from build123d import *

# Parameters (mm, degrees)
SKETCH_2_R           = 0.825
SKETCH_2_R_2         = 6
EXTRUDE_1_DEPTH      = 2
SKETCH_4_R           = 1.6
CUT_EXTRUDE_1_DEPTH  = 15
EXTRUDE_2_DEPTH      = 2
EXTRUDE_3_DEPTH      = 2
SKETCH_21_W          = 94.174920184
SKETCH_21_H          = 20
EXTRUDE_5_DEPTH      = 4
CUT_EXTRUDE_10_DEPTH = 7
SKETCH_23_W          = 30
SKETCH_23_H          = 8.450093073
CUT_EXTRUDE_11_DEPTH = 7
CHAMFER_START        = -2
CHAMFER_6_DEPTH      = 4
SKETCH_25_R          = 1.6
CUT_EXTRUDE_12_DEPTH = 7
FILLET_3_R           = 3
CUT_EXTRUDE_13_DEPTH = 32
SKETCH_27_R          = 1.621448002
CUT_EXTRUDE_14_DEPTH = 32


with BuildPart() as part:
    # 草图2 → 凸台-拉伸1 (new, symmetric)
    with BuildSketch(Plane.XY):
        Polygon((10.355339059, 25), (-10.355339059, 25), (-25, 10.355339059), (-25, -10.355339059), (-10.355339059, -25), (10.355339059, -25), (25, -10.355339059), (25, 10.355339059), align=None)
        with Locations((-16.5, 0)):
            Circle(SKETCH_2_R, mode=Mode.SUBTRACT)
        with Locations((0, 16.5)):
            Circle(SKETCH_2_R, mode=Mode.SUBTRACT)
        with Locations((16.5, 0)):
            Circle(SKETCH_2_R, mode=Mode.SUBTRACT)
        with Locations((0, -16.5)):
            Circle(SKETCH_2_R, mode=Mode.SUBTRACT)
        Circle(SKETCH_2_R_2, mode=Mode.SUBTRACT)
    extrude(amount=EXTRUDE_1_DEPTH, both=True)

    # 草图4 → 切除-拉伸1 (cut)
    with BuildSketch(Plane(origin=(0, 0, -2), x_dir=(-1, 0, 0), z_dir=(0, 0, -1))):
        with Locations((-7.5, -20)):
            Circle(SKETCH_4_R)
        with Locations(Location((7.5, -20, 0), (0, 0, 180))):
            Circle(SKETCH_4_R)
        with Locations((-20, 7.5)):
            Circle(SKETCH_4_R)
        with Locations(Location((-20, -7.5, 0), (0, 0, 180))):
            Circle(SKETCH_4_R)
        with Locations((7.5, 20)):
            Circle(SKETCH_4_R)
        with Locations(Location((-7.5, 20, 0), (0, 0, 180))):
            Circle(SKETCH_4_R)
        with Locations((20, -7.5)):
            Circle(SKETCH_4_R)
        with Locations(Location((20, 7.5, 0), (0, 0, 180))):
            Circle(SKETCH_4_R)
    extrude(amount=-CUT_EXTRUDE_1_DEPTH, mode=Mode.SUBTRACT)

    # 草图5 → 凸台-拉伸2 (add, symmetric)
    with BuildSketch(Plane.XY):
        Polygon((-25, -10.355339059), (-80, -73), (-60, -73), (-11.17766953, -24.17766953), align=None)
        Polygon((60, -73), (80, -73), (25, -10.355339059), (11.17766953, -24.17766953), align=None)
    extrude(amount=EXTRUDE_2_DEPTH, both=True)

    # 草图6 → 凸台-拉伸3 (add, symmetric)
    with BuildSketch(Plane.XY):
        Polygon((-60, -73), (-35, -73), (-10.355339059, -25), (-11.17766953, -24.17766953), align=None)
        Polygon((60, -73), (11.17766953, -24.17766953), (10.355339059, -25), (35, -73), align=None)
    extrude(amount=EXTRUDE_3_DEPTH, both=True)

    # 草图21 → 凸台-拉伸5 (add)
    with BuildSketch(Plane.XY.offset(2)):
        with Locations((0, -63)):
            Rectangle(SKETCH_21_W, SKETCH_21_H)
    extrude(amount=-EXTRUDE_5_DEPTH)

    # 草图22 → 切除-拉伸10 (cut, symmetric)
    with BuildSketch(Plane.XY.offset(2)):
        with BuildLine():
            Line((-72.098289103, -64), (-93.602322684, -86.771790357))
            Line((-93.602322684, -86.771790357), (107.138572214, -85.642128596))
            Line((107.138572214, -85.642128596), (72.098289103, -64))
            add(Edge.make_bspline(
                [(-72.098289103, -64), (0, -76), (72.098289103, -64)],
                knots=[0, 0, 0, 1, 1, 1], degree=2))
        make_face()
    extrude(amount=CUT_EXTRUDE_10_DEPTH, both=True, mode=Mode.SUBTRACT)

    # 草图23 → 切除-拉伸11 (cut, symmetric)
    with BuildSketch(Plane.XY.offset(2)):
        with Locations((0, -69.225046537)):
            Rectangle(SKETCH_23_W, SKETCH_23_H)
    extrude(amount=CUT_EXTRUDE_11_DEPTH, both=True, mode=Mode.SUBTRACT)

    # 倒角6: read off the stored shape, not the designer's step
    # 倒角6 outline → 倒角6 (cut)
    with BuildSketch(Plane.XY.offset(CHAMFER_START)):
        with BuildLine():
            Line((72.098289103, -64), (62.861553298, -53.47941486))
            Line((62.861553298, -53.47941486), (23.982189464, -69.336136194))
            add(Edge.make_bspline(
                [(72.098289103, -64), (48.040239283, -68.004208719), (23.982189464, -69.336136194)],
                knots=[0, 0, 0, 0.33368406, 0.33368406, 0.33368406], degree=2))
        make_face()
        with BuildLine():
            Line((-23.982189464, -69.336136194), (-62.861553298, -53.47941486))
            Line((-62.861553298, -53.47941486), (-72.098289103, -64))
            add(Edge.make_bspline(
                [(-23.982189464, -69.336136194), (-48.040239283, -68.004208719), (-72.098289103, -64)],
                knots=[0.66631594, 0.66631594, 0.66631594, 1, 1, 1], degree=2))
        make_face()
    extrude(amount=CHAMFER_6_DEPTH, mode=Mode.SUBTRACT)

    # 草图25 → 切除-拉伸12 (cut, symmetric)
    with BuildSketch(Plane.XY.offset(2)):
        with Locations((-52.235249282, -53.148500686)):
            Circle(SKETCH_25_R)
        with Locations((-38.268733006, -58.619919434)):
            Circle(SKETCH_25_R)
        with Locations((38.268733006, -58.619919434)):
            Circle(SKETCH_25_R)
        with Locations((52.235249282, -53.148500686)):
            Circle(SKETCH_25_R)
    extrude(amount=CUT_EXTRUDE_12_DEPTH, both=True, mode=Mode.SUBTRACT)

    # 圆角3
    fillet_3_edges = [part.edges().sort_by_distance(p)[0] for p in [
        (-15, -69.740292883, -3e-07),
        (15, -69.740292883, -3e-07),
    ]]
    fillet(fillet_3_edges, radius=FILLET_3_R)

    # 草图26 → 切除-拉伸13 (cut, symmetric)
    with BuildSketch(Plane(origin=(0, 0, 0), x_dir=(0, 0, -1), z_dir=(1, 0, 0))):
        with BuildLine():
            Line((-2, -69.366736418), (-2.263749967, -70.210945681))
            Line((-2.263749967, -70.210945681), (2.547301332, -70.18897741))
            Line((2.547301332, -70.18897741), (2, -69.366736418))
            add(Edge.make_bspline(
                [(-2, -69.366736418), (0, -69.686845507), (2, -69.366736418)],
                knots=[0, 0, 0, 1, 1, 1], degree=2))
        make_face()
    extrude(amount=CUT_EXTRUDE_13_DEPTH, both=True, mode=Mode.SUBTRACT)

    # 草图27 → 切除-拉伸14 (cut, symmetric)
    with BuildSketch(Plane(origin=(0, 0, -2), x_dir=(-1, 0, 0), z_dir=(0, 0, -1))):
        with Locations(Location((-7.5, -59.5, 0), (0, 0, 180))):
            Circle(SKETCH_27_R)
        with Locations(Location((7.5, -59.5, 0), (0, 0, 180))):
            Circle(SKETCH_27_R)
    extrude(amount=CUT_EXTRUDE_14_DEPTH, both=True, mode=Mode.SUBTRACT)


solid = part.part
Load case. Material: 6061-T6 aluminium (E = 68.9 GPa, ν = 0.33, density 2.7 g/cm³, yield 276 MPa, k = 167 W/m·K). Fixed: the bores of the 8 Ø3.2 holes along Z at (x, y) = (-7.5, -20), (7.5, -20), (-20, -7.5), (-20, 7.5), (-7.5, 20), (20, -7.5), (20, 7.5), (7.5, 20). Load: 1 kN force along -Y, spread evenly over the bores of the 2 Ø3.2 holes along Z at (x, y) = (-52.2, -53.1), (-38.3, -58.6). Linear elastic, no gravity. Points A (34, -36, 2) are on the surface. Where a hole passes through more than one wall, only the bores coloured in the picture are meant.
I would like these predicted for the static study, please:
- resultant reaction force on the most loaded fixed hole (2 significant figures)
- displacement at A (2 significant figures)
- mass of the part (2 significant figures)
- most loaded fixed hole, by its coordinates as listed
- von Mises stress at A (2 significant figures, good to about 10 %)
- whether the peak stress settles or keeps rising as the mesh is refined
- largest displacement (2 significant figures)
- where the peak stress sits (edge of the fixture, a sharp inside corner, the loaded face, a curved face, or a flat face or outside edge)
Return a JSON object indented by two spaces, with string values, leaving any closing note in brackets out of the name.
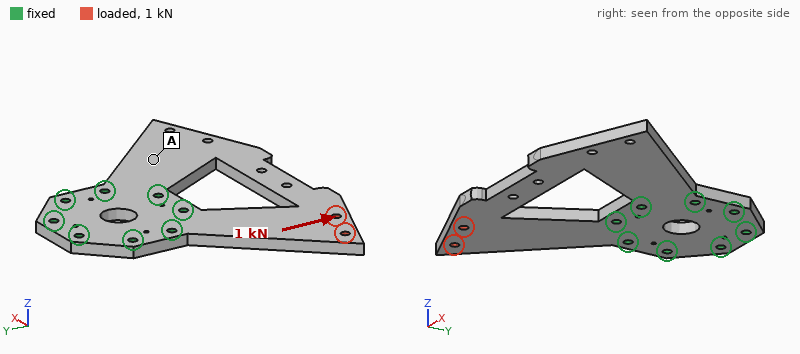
{
  "resultant reaction force on the most loaded fixed hole": "1.3 kN",
  "displacement at A": "20 µm",
  "mass of the part": "58 g",
  "most loaded fixed hole, by its coordinates as listed": "(-20, -7.5)",
  "von Mises stress at A": "7.6 MPa",
  "whether the peak stress settles or keeps rising as the mesh is refined": "keeps rising",
  "largest displacement": "73 µm",
  "where the peak stress sits": "a sharp inside corner"
}
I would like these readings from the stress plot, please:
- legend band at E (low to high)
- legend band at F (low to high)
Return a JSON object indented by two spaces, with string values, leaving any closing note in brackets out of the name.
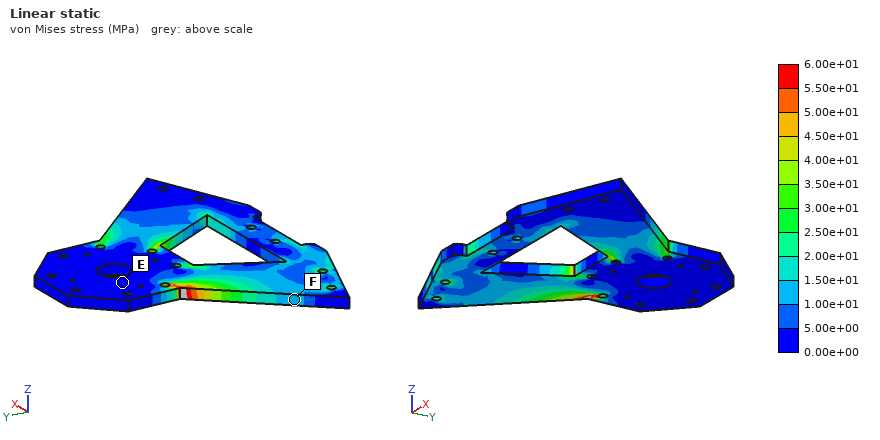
{
  "legend band at E": "0.00e+00 to 5.00e+00 MPa",
  "legend band at F": "1.00e+01 to 1.50e+01 MPa"
}
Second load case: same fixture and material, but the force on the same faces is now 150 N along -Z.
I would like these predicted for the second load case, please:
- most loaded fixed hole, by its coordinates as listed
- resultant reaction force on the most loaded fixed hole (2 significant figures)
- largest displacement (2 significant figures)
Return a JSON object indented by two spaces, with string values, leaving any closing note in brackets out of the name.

{
  "most loaded fixed hole, by its coordinates as listed": "(-7.5, -20)",
  "resultant reaction force on the most loaded fixed hole": "170 N",
  "largest displacement": "0.86 mm"
}
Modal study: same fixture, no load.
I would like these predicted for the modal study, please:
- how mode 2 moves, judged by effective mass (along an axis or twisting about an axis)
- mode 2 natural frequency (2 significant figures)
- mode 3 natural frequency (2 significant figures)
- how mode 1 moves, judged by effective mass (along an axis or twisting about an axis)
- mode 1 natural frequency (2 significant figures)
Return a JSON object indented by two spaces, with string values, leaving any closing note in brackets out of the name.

{
  "how mode 2 moves, judged by effective mass": "twisting about Y",
  "mode 2 natural frequency": "940 Hz",
  "mode 3 natural frequency": "2100 Hz",
  "how mode 1 moves, judged by effective mass": "along Z",
  "mode 1 natural frequency": "780 Hz"
}
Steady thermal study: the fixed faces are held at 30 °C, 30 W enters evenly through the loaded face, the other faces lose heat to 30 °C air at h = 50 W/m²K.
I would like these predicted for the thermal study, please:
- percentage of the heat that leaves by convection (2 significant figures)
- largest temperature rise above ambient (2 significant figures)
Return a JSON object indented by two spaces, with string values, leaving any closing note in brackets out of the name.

{
  "percentage of the heat that leaves by convection": "33 %",
  "largest temperature rise above ambient": "68 K"
}
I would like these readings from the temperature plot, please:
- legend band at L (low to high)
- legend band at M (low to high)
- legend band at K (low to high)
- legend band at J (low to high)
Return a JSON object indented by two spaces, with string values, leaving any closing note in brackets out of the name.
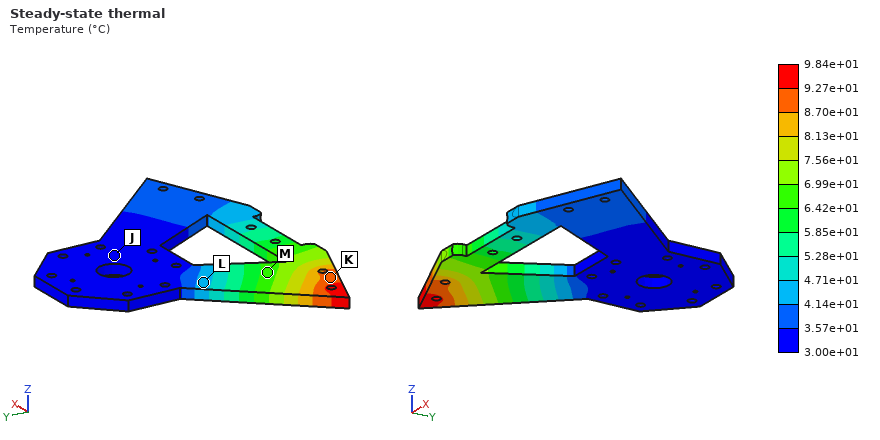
{
  "legend band at L": "4.14e+01 to 4.71e+01 °C",
  "legend band at M": "6.42e+01 to 6.99e+01 °C",
  "legend band at K": "8.70e+01 to 9.27e+01 °C",
  "legend band at J": "3.00e+01 to 3.57e+01 °C"
}
